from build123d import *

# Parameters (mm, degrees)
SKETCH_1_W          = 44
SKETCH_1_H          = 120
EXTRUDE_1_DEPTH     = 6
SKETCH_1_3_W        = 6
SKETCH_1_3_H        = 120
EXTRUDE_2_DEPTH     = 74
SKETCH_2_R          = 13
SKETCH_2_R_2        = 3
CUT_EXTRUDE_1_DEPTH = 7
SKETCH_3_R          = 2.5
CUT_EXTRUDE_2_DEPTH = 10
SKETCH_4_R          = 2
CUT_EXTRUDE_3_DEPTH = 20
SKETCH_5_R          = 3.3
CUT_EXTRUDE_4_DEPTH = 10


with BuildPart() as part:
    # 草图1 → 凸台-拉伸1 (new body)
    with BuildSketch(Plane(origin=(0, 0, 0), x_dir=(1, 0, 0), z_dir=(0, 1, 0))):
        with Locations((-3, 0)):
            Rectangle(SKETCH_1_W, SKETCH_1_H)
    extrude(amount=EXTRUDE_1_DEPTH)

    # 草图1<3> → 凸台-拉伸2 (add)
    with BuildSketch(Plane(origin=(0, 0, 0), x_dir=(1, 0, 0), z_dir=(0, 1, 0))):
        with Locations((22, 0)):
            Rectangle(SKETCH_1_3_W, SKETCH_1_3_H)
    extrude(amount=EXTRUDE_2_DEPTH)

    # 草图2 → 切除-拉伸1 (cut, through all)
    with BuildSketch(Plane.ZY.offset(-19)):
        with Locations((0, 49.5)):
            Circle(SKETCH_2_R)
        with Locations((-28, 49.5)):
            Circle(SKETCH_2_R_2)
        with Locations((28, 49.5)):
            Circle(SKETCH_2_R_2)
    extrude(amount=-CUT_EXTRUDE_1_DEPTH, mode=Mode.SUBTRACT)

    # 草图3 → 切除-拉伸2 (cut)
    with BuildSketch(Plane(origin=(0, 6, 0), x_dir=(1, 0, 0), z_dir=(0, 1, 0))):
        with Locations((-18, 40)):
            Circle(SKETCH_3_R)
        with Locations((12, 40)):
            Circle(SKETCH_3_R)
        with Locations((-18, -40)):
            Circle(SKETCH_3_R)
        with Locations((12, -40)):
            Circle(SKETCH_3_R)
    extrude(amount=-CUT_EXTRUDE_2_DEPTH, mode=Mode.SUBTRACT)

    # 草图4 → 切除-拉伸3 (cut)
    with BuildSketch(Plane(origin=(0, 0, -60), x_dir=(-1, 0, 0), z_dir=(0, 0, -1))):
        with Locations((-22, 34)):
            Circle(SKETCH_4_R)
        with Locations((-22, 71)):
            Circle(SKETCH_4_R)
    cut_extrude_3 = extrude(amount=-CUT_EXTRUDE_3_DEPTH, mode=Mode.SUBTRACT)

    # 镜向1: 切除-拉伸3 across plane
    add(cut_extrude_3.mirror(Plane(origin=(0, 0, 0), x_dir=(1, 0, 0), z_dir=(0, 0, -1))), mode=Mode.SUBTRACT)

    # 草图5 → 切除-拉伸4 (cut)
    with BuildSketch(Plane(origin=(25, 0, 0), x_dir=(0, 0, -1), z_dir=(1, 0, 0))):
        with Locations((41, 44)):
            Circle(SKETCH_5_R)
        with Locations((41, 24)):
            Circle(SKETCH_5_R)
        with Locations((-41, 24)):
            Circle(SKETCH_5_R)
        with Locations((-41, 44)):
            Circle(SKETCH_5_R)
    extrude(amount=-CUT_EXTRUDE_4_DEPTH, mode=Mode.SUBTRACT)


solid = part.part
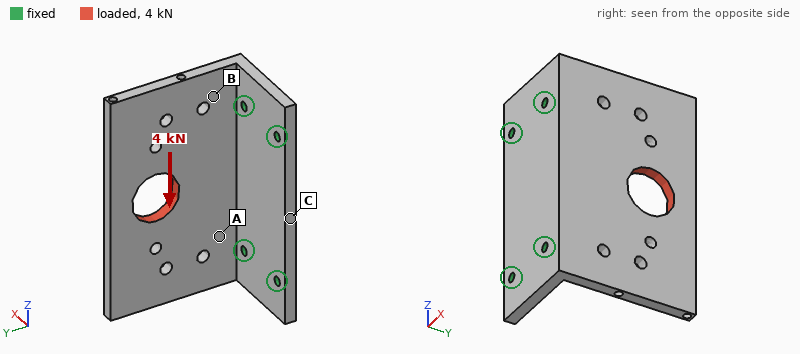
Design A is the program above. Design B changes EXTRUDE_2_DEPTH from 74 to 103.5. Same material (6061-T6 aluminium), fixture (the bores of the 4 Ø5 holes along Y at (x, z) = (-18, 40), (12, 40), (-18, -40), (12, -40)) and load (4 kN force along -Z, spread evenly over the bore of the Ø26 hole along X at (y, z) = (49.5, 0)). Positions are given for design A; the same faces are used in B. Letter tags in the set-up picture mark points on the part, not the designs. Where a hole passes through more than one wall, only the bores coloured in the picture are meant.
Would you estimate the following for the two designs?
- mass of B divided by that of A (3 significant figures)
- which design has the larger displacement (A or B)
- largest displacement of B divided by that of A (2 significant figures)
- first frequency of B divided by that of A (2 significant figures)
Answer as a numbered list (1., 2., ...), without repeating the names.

1. 1.27
2. B
3. 1.1
4. 0.49
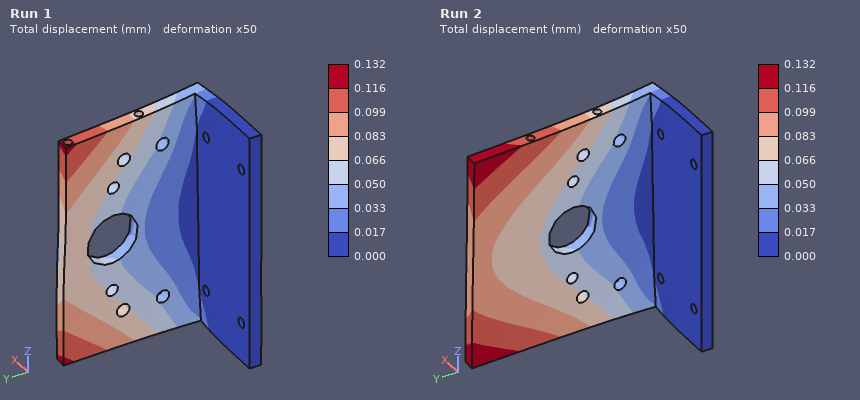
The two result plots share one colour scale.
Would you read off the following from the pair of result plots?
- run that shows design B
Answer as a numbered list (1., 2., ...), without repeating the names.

1. Run 2
